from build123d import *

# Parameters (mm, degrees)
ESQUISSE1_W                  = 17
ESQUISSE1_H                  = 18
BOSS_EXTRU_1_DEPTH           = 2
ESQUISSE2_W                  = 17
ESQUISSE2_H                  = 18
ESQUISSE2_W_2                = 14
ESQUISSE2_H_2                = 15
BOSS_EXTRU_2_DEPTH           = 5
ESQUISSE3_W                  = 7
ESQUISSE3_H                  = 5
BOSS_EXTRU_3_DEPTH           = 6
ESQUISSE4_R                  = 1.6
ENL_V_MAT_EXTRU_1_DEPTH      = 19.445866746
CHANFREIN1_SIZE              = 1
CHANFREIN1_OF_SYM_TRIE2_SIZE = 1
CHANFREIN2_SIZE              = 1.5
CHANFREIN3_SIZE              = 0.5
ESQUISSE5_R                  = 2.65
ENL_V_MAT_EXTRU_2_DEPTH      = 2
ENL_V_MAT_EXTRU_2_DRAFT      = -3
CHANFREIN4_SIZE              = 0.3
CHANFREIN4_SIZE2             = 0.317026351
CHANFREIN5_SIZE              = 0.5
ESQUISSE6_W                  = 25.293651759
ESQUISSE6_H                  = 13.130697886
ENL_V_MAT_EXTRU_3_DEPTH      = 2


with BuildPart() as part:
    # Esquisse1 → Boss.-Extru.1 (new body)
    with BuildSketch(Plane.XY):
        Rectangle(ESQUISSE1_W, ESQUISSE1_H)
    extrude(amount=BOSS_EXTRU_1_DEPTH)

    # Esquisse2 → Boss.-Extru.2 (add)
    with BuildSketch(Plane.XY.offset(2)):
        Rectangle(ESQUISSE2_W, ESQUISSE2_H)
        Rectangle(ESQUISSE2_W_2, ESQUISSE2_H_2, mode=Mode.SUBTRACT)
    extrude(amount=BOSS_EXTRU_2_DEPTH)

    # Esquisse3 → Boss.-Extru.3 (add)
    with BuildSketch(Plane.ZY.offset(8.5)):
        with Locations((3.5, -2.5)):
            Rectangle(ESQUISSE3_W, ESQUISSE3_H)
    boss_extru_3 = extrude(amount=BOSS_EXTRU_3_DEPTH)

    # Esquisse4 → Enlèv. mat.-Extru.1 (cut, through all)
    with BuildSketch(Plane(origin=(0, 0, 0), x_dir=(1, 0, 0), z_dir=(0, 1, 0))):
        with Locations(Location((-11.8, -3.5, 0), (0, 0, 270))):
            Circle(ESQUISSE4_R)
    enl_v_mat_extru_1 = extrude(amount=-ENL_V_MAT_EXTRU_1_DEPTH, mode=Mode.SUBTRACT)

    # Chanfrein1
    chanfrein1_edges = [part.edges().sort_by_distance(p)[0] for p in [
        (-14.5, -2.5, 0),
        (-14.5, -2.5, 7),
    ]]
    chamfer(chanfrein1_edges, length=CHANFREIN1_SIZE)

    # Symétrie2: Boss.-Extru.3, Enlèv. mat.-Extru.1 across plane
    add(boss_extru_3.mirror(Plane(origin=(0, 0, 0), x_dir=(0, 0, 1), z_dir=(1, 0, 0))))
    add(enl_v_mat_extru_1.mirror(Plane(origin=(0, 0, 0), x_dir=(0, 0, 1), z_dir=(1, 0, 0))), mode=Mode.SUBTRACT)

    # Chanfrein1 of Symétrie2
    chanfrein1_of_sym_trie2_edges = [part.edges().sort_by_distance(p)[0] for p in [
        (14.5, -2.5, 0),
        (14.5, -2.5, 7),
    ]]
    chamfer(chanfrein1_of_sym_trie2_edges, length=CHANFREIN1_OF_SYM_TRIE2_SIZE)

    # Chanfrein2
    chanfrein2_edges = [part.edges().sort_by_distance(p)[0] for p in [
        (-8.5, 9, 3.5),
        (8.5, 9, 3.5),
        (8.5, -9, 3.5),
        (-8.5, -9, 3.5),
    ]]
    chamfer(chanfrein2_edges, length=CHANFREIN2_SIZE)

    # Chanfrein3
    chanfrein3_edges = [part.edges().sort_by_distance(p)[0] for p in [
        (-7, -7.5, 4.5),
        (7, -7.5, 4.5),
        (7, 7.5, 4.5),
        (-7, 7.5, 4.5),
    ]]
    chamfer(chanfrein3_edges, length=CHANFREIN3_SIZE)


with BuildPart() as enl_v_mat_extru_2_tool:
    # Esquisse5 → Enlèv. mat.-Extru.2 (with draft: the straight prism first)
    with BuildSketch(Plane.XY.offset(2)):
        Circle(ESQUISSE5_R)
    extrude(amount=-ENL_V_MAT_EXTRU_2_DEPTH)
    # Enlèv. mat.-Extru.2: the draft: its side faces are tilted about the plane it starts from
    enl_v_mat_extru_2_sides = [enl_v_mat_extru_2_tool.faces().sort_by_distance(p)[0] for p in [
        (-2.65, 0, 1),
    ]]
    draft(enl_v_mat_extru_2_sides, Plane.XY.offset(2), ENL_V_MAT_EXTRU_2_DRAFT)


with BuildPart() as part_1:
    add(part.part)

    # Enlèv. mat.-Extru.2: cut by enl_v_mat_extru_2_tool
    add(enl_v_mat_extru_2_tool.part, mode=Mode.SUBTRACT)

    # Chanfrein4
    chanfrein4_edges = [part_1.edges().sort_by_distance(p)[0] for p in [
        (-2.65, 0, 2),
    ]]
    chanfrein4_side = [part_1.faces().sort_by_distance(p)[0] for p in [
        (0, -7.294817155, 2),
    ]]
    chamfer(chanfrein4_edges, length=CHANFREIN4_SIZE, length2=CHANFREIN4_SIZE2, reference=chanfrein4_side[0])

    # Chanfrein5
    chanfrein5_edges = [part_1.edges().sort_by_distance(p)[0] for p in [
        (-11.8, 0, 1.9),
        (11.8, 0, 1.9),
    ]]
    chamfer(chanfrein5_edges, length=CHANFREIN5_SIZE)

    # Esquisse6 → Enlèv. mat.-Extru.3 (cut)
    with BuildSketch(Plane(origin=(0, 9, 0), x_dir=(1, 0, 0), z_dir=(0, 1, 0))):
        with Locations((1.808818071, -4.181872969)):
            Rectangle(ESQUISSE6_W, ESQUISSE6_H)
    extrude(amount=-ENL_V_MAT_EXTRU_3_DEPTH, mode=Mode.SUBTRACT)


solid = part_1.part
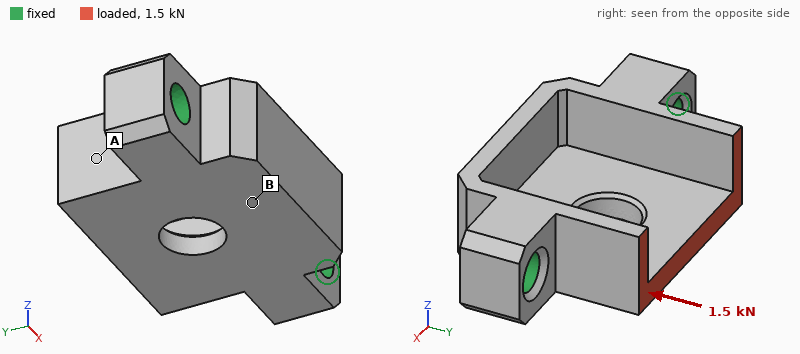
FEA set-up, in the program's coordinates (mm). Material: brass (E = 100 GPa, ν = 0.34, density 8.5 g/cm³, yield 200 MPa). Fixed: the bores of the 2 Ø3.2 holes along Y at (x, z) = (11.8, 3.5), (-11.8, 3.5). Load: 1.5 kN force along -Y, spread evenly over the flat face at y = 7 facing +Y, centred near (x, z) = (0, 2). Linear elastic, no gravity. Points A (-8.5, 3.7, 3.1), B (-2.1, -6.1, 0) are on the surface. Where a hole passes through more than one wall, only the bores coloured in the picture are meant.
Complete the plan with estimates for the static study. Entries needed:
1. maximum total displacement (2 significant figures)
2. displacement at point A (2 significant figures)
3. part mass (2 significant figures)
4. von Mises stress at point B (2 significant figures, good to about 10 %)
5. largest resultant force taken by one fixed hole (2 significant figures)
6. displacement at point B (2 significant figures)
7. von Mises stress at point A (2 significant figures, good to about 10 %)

14 µm
6.3 µm
9.8 g
17 MPa
750 N
6.9 µm
34 MPa
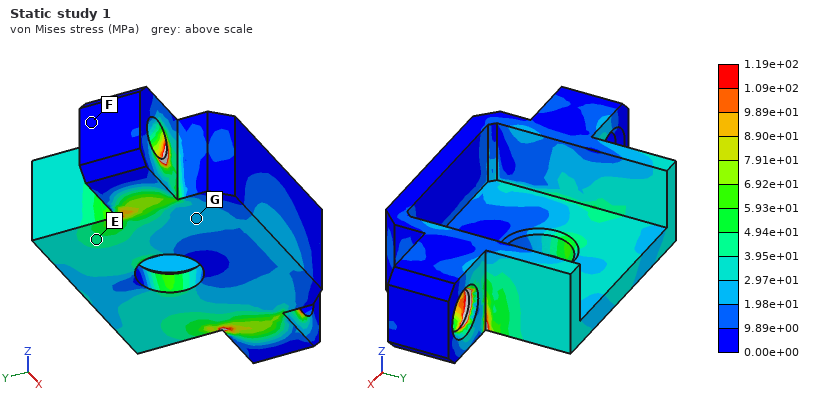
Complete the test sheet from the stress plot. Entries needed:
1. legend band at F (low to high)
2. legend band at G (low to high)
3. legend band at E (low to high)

0.00e+00 to 9.89e+00 MPa
1.98e+01 to 2.97e+01 MPa
3.95e+01 to 4.94e+01 MPa
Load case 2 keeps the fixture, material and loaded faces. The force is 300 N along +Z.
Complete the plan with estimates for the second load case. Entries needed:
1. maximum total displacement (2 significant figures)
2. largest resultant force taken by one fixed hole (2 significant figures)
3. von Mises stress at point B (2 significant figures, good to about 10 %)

31 µm
170 N
9.9 MPa
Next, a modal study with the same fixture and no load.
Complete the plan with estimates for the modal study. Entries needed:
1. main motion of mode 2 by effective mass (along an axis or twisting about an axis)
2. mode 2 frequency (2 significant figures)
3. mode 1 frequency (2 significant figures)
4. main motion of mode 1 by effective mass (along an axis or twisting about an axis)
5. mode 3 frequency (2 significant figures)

along Z
22 kHz
16 kHz
along Z
23 kHz
